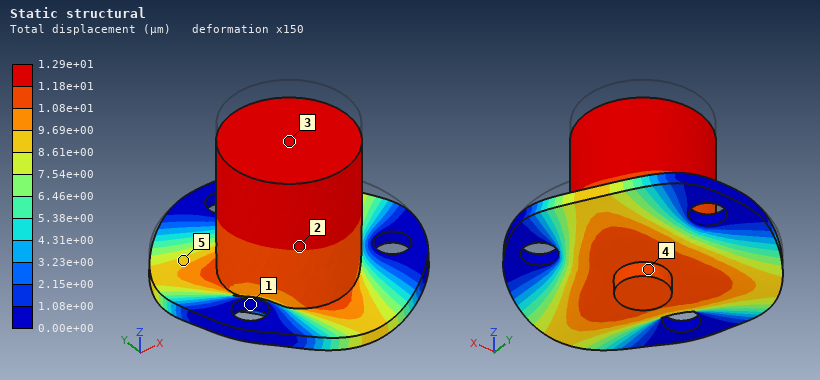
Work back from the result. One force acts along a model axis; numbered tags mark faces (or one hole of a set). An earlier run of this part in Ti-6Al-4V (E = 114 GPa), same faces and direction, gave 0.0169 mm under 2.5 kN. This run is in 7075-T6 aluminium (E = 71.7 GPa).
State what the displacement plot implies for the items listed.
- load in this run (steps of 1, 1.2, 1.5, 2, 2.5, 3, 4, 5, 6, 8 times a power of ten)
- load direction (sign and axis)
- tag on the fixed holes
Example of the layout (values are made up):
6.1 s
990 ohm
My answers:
1.2 kN
-Z
1
